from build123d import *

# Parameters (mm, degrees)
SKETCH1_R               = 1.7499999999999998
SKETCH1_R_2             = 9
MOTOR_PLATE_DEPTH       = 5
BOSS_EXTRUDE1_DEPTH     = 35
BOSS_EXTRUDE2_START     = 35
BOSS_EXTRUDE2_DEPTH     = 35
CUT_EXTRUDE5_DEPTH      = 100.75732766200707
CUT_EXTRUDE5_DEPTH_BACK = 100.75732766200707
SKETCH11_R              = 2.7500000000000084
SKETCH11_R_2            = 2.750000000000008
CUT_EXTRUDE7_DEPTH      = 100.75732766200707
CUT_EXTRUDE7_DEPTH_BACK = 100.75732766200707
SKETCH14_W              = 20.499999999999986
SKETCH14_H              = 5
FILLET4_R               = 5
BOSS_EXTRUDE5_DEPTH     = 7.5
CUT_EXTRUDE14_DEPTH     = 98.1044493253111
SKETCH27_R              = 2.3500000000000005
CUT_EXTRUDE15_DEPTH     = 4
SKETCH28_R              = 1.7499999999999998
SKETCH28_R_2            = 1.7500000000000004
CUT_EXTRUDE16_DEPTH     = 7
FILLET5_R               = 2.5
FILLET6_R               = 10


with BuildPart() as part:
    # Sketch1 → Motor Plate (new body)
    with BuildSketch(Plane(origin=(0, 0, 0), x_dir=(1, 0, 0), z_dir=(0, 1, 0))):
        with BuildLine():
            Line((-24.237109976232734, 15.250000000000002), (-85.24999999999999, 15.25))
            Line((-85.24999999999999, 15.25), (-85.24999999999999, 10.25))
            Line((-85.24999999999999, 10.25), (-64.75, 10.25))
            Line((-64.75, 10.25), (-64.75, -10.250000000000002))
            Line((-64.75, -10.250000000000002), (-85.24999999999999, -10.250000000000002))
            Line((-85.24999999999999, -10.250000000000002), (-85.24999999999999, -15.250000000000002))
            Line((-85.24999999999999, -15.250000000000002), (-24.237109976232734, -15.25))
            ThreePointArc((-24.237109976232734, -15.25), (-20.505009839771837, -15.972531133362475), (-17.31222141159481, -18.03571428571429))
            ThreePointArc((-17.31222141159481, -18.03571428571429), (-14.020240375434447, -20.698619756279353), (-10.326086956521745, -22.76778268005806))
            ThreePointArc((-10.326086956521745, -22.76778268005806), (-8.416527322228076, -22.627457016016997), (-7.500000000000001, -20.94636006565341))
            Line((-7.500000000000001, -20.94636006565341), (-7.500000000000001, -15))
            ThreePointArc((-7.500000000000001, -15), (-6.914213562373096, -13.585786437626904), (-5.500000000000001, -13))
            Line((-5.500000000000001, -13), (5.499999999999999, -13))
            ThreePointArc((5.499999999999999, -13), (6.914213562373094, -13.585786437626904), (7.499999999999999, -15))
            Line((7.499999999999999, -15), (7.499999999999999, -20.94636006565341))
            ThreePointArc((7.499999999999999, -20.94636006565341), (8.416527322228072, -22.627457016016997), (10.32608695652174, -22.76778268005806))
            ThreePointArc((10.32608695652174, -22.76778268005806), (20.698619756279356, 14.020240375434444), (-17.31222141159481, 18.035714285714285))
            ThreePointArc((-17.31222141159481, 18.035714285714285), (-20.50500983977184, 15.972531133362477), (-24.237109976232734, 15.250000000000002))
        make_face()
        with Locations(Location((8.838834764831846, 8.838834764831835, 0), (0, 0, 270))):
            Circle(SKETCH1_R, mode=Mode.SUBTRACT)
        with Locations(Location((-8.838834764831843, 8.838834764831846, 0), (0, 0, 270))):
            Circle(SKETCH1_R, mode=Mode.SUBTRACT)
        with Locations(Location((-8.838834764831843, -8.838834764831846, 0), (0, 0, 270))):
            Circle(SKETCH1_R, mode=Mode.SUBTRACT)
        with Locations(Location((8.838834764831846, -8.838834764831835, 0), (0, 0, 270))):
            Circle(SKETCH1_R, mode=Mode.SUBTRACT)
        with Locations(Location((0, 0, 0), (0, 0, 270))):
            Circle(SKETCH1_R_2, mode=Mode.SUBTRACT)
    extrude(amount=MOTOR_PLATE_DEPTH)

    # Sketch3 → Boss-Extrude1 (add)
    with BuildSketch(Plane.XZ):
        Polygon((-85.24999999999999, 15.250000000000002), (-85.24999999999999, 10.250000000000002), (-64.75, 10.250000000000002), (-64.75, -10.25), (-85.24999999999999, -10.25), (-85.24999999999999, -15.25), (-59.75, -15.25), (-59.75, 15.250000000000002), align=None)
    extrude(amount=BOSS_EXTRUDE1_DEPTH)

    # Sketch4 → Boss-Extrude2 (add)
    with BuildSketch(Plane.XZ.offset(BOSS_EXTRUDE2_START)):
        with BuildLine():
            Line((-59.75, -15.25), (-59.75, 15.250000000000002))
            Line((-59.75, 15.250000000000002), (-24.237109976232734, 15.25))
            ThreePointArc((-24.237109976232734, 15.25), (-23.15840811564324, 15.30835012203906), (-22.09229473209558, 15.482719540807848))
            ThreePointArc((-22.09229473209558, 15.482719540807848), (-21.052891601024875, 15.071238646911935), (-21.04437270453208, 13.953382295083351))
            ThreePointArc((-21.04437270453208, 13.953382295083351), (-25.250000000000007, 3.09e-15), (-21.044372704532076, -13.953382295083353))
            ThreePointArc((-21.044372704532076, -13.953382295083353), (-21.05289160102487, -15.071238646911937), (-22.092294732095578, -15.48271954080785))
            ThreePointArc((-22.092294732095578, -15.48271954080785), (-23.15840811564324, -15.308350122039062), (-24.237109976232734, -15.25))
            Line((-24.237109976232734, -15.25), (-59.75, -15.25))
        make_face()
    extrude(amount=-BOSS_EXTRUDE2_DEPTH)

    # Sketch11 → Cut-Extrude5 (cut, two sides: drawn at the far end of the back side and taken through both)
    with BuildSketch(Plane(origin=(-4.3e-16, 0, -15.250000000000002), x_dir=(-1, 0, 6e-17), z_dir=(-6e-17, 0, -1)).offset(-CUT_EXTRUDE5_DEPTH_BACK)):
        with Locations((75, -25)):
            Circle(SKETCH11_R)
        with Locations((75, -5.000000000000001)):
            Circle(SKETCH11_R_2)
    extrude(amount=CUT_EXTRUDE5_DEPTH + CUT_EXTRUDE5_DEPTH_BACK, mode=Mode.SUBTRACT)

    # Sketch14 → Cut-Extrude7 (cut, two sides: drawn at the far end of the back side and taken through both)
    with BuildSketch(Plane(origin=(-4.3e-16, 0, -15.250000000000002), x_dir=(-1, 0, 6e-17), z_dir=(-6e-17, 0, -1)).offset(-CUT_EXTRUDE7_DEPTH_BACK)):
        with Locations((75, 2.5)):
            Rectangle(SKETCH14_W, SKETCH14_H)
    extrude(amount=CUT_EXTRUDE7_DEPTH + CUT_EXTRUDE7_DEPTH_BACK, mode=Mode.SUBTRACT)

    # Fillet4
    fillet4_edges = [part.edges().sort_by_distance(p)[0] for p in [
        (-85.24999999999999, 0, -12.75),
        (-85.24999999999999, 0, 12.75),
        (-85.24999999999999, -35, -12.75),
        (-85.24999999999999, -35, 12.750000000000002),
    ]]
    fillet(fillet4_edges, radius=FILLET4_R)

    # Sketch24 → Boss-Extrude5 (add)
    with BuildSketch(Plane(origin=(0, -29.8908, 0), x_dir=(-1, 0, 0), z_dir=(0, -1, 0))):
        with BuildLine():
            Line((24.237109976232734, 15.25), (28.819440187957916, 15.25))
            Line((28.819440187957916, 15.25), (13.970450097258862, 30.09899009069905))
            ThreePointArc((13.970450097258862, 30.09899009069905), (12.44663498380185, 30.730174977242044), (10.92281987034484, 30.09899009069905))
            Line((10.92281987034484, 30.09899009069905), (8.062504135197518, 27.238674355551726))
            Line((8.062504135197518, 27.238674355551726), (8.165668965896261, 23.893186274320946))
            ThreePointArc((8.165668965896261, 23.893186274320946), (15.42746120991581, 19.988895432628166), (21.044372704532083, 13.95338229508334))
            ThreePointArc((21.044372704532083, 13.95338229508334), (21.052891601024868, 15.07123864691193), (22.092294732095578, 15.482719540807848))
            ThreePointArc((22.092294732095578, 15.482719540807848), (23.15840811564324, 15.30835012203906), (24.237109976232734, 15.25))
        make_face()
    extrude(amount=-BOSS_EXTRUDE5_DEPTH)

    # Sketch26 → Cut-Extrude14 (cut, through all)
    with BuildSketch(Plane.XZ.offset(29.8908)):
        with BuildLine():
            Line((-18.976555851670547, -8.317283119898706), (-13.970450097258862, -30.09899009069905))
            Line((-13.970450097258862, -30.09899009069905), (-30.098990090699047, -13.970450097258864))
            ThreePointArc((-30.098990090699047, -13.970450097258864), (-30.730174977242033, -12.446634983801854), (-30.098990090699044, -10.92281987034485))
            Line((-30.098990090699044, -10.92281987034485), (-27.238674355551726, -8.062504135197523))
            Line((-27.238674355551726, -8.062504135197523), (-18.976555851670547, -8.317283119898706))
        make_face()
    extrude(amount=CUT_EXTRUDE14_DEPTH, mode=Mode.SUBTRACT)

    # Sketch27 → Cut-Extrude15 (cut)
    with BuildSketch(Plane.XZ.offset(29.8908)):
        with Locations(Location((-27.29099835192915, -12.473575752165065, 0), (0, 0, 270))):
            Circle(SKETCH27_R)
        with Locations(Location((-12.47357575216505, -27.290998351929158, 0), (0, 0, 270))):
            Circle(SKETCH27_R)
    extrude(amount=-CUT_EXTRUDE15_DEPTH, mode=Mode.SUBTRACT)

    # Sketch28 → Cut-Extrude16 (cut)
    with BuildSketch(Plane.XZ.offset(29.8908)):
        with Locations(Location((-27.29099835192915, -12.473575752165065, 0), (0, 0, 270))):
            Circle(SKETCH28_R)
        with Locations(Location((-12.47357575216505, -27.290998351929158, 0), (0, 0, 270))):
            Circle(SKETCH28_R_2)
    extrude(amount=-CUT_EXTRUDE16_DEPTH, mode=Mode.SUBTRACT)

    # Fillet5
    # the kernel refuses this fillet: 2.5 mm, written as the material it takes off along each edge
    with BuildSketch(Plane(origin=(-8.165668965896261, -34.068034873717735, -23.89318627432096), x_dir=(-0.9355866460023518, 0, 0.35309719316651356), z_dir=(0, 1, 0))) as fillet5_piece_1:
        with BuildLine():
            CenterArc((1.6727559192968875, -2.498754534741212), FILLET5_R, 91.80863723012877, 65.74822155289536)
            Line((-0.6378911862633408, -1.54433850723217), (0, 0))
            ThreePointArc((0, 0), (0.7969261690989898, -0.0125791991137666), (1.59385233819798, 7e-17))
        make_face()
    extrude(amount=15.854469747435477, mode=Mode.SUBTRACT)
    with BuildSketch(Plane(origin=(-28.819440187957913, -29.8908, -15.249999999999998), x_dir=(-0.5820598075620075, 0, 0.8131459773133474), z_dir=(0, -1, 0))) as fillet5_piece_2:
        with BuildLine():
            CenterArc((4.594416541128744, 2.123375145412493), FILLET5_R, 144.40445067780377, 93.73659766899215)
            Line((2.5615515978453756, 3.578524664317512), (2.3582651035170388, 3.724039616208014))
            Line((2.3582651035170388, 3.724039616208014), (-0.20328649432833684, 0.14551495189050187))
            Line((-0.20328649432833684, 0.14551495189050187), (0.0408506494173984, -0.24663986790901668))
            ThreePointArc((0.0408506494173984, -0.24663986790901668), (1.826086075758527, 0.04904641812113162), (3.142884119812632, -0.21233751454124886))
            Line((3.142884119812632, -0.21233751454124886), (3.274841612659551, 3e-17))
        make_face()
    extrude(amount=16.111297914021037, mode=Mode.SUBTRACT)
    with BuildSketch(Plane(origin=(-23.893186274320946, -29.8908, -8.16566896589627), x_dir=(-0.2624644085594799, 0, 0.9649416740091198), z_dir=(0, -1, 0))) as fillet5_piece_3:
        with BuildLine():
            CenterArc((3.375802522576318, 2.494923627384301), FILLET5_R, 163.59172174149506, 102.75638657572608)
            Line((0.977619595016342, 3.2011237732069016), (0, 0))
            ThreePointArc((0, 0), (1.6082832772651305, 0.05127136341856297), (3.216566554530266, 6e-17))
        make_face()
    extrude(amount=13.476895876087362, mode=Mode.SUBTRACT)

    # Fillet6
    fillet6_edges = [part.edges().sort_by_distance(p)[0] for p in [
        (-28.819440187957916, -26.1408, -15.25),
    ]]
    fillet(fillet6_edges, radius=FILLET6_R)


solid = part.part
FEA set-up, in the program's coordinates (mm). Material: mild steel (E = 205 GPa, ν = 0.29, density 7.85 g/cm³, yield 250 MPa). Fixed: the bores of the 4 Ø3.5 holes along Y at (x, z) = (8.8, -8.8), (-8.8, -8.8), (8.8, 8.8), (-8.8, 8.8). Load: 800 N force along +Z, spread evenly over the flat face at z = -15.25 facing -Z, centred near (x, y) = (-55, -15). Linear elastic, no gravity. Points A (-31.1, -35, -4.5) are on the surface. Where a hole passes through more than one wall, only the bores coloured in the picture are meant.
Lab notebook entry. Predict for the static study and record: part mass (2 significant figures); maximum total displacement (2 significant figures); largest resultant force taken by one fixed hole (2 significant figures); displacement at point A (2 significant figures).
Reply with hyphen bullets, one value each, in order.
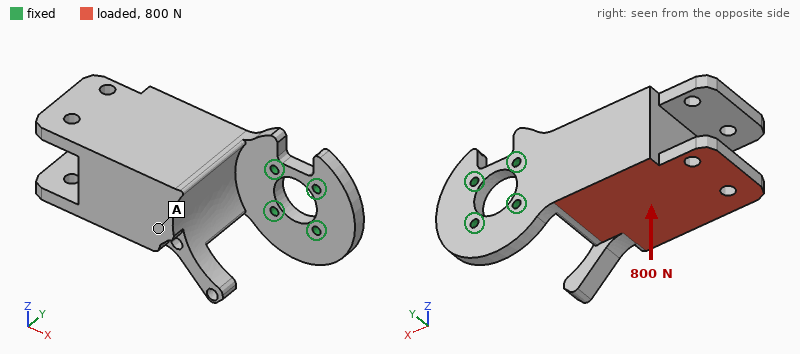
- 510 g
- 47 µm
- 1.6 kN
- 30 µm
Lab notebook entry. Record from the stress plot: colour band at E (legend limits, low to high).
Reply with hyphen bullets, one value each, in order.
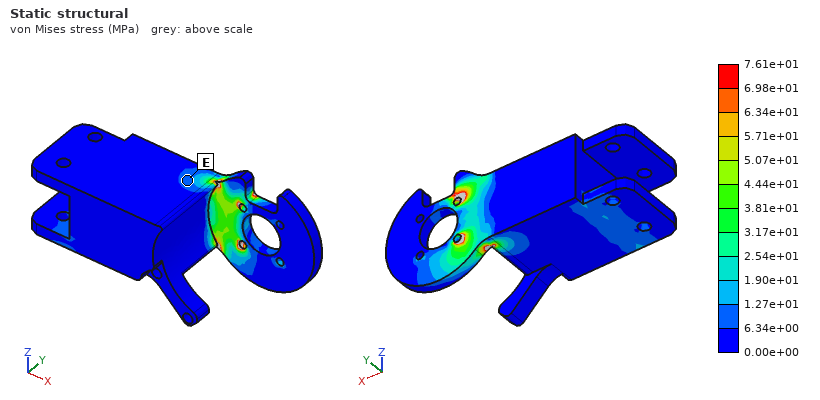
- 6.34e+00 to 1.27e+01 MPa
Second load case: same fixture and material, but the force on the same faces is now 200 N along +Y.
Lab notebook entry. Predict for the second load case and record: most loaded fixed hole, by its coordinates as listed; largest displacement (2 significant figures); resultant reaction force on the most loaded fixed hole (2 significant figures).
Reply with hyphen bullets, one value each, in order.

- (-8.8, -8.8)
- 0.14 mm
- 300 N
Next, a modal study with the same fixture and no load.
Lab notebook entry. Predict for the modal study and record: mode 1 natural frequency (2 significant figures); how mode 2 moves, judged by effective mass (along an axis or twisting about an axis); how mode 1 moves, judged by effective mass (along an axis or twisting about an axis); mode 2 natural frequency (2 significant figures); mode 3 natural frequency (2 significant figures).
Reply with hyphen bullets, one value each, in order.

- 380 Hz
- along Z
- along Y
- 1300 Hz
- 3000 Hz
